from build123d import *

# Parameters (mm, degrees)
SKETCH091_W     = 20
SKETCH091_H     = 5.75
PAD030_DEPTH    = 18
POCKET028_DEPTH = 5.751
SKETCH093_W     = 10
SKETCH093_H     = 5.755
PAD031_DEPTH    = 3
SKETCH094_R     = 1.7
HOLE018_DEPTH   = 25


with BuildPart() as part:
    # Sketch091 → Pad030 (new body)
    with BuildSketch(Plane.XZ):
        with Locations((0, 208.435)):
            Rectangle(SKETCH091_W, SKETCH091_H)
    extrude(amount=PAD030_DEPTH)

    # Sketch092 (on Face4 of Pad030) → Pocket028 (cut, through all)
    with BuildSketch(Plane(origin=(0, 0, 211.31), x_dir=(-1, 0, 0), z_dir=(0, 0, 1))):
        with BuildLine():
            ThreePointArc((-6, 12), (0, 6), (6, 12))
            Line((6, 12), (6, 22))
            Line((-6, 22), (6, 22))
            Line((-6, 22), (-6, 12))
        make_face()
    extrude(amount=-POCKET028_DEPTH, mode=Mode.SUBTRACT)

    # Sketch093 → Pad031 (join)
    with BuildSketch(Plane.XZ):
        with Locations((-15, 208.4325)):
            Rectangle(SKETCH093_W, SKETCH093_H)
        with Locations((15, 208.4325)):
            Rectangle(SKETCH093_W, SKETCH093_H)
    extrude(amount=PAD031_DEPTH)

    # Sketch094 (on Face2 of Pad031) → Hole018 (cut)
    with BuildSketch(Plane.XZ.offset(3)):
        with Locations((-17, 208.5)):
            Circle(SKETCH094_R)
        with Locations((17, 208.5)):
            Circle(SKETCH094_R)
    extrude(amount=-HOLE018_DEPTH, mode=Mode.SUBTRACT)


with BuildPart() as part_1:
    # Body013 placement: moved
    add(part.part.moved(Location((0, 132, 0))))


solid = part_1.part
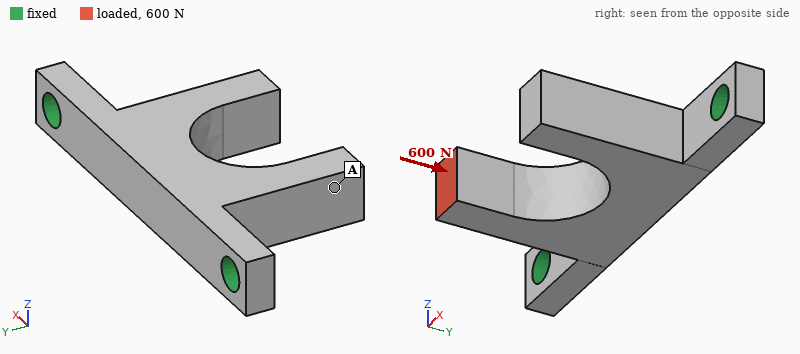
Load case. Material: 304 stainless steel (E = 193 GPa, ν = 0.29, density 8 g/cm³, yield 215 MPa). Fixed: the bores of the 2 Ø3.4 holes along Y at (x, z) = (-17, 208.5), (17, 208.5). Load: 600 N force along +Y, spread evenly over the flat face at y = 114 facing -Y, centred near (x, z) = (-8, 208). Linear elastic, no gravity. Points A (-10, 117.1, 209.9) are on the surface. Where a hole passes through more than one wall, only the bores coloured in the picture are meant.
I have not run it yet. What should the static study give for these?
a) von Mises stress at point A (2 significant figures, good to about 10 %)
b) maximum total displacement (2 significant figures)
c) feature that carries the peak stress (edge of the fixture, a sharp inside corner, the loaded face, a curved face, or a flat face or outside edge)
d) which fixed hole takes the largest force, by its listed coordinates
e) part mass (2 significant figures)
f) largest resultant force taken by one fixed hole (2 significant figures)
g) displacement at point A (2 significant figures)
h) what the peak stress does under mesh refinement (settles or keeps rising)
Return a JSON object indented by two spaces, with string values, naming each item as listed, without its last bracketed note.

{
  "von Mises stress at point A": "26 MPa",
  "maximum total displacement": "12 µm",
  "feature that carries the peak stress": "edge of the fixture",
  "which fixed hole takes the largest force, by its listed coordinates": "(-17, 208.5)",
  "part mass": "13 g",
  "largest resultant force taken by one fixed hole": "520 N",
  "displacement at point A": "11 µm",
  "what the peak stress does under mesh refinement": "keeps rising"
}
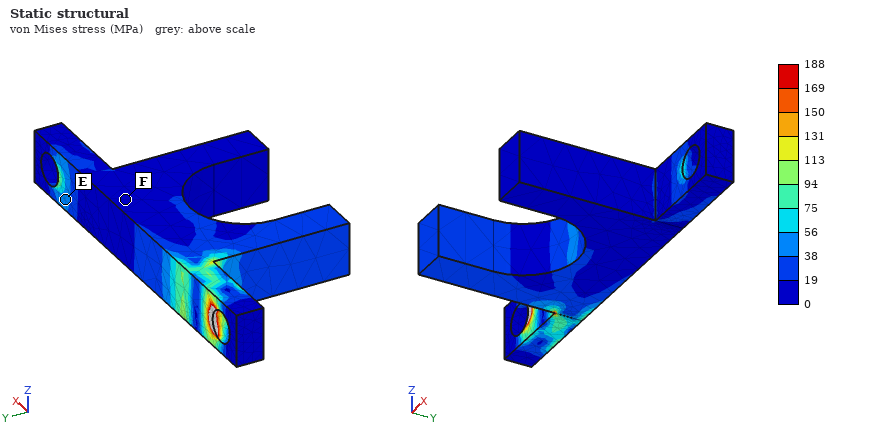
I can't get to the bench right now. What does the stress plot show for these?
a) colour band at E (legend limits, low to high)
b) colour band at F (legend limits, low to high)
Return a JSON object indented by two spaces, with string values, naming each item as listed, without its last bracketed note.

{
  "colour band at E": "38 to 56 MPa",
  "colour band at F": "0 to 19 MPa"
}
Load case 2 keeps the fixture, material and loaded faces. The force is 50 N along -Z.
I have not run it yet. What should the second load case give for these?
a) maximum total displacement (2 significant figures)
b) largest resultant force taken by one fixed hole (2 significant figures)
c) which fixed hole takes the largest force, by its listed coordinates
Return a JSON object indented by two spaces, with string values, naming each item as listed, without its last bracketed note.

{
  "maximum total displacement": "23 µm",
  "largest resultant force taken by one fixed hole": "40 N",
  "which fixed hole takes the largest force, by its listed coordinates": "(-17, 208.5)"
}
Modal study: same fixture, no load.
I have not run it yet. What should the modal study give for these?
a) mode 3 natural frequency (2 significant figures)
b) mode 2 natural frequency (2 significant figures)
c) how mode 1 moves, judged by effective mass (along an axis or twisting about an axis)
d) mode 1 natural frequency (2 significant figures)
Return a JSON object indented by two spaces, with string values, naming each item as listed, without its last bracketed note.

{
  "mode 3 natural frequency": "13 kHz",
  "mode 2 natural frequency": "13 kHz",
  "how mode 1 moves, judged by effective mass": "along Z",
  "mode 1 natural frequency": "5500 Hz"
}
